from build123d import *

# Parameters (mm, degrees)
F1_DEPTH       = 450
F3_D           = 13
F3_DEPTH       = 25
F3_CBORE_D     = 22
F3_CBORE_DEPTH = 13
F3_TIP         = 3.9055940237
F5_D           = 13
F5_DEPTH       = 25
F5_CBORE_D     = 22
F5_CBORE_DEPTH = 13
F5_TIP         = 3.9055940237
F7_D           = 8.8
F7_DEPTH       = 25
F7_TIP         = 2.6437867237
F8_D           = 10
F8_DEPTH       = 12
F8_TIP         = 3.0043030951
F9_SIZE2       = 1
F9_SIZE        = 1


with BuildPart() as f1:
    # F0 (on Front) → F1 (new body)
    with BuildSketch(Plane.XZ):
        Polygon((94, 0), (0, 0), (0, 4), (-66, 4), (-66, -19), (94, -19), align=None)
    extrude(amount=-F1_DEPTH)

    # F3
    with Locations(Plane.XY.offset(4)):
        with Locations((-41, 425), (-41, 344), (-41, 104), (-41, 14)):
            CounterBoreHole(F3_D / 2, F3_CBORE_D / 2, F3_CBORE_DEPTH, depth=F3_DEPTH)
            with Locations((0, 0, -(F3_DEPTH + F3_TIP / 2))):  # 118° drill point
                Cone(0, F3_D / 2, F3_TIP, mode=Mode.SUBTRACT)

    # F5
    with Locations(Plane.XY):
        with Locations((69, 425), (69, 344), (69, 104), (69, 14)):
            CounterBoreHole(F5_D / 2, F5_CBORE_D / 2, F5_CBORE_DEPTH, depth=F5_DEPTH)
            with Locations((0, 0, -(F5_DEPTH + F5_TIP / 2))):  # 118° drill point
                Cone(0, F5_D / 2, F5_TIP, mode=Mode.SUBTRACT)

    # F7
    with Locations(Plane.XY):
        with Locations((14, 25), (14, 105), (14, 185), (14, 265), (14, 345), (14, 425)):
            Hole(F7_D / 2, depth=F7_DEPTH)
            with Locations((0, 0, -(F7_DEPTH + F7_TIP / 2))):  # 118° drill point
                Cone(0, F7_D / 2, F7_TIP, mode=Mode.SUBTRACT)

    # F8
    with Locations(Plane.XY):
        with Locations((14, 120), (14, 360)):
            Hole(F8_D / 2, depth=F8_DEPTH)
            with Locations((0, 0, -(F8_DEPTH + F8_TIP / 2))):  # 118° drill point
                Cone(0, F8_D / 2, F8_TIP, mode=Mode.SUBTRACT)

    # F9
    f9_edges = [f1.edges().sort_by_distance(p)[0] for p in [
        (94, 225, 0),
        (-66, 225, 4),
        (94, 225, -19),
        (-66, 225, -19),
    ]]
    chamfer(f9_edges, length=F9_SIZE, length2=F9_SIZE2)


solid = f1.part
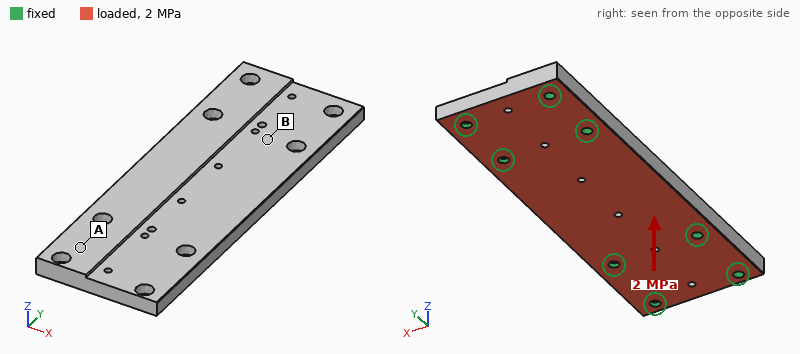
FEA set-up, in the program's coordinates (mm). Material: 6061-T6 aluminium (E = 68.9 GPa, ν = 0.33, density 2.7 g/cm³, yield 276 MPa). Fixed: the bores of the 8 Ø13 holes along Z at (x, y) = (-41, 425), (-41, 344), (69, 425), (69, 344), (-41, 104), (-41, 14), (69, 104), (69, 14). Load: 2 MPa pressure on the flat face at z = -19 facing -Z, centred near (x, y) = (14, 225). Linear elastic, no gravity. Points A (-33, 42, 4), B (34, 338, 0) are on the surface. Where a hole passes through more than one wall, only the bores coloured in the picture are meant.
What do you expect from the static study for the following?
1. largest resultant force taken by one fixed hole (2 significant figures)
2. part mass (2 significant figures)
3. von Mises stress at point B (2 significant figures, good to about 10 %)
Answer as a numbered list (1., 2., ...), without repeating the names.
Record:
1. 37 kN
2. 3.9 kg
3. 78 MPa
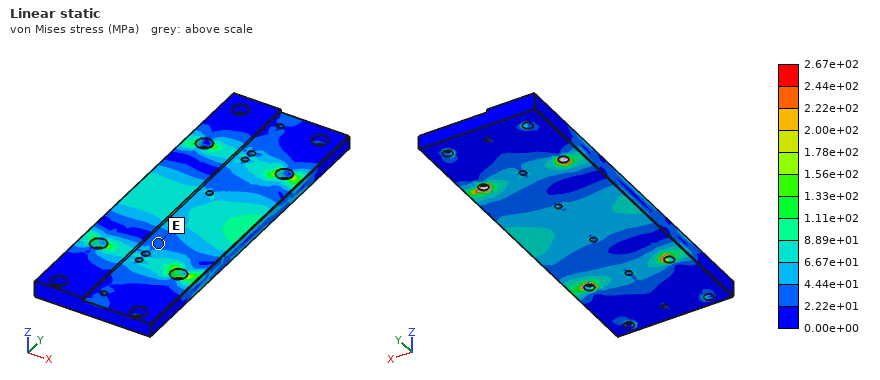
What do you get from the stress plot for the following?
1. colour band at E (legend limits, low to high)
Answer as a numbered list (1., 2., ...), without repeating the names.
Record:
1. 2.22e+01 to 4.44e+01 MPa
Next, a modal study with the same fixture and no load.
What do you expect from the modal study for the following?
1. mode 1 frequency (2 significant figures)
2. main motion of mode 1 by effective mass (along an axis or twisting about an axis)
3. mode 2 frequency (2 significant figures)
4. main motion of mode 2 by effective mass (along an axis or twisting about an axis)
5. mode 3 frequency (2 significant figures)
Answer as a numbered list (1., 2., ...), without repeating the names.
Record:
1. 1400 Hz
2. along Z
3. 2200 Hz
4. twisting about Y
5. 3700 Hz
